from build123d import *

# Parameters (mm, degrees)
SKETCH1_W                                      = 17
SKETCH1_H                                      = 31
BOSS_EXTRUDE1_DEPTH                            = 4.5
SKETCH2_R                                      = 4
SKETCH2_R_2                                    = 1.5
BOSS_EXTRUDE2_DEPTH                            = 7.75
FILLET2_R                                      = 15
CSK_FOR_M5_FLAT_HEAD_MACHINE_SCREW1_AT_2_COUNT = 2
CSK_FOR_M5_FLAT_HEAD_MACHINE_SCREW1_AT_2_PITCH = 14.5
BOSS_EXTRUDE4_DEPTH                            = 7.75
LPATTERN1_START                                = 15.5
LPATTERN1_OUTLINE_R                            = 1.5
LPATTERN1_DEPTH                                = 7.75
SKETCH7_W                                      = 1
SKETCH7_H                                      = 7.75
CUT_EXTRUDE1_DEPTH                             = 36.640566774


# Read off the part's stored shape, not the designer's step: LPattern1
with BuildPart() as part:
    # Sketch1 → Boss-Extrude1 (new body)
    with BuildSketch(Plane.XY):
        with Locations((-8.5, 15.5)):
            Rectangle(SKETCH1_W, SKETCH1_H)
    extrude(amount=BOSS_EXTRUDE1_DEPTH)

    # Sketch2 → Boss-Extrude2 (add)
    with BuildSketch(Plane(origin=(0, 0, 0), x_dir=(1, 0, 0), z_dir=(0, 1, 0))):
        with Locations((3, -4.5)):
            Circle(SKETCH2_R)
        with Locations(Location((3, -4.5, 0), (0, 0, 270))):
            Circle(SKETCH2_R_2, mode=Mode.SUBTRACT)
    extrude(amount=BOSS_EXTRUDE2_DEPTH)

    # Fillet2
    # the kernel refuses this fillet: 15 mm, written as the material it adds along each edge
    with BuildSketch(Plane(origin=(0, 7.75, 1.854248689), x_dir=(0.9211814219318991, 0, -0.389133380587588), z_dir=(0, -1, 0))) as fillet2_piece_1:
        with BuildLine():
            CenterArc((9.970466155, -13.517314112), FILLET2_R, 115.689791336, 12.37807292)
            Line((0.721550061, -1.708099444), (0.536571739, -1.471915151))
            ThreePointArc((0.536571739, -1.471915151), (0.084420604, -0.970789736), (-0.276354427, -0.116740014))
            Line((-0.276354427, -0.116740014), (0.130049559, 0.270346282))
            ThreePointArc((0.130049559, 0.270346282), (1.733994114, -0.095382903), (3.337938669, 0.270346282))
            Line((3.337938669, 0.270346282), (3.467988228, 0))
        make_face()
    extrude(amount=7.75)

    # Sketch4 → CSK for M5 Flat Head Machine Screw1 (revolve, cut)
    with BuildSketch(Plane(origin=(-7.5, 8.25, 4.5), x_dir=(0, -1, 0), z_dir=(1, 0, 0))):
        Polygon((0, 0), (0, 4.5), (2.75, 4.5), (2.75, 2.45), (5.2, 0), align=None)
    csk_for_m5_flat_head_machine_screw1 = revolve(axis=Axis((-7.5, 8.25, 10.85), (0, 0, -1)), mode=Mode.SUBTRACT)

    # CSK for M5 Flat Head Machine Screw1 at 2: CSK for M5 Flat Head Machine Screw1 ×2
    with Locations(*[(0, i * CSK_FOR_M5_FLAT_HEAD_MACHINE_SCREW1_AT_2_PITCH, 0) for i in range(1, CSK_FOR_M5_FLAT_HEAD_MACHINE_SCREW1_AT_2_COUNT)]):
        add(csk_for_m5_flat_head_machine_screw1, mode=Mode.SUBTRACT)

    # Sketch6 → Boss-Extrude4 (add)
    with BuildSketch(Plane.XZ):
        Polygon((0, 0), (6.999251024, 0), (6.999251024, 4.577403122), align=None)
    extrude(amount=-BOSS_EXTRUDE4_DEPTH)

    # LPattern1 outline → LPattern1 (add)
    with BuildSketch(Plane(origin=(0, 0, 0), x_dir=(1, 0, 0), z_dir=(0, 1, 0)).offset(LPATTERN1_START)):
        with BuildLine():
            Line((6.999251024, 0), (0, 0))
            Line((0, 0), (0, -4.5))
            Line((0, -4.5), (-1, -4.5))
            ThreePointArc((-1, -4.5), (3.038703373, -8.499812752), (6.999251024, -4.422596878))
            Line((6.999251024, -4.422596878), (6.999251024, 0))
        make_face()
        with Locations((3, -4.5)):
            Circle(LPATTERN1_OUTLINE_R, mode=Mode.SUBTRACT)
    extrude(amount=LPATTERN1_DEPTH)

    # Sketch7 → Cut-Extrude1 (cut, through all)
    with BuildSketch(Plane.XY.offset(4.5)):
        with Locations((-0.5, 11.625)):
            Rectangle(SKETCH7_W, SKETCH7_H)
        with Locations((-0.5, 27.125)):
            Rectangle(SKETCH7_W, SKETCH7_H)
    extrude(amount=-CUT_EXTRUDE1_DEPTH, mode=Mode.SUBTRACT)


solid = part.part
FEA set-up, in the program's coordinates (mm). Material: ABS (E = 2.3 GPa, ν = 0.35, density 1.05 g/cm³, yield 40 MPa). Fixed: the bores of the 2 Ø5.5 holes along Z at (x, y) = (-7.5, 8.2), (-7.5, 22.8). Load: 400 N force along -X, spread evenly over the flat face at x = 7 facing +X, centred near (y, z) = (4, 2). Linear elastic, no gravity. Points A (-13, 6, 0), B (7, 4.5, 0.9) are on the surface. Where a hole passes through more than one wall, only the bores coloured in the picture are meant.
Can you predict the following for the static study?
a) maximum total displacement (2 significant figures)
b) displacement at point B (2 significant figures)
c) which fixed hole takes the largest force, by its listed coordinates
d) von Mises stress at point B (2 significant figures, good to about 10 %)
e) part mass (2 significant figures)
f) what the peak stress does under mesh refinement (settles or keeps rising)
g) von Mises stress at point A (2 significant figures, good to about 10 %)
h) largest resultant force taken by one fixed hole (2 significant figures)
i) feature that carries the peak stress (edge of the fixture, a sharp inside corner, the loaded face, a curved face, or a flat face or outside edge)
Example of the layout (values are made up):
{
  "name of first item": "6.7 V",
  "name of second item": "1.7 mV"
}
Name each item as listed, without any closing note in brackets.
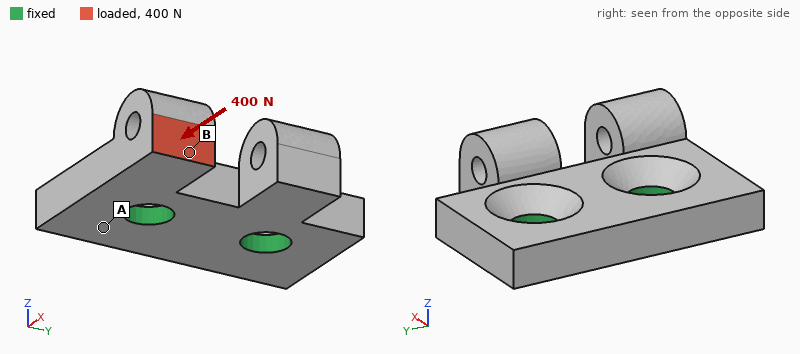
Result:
{
  "maximum total displacement": "0.26 mm",
  "displacement at point B": "0.21 mm",
  "which fixed hole takes the largest force, by its listed coordinates": "(-7.5, 8.2)",
  "von Mises stress at point B": "11 MPa",
  "part mass": "2.9 g",
  "what the peak stress does under mesh refinement": "keeps rising",
  "von Mises stress at point A": "5.6 MPa",
  "largest resultant force taken by one fixed hole": "440 N",
  "feature that carries the peak stress": "edge of the fixture"
}
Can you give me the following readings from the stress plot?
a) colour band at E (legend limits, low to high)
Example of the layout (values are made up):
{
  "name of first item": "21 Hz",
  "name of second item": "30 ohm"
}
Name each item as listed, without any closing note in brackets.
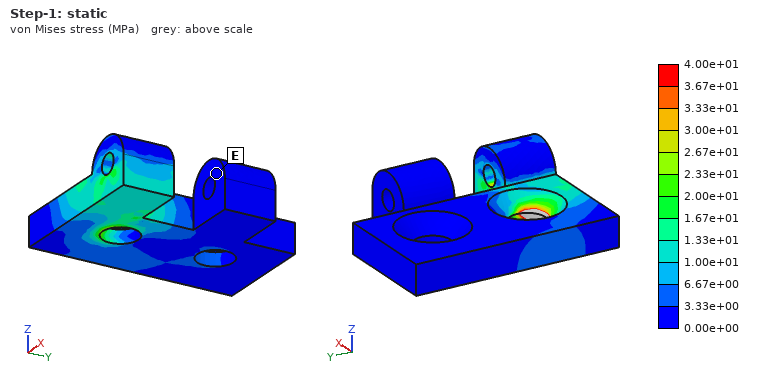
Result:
{
  "colour band at E": "0.00e+00 to 3.33e+00 MPa"
}
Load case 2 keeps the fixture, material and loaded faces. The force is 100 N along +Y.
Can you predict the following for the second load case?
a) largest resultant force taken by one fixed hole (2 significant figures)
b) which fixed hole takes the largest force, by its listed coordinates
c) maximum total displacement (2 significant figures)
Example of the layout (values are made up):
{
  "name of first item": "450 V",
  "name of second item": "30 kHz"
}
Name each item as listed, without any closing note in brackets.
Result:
{
  "largest resultant force taken by one fixed hole": "92 N",
  "which fixed hole takes the largest force, by its listed coordinates": "(-7.5, 8.2)",
  "maximum total displacement": "0.26 mm"
}
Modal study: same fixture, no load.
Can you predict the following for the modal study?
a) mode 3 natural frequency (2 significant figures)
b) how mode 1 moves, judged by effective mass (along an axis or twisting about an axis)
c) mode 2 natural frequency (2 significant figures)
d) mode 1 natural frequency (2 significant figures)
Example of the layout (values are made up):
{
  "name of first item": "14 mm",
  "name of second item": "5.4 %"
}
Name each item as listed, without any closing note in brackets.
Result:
{
  "mode 3 natural frequency": "6600 Hz",
  "how mode 1 moves, judged by effective mass": "along Z",
  "mode 2 natural frequency": "4000 Hz",
  "mode 1 natural frequency": "3300 Hz"
}
